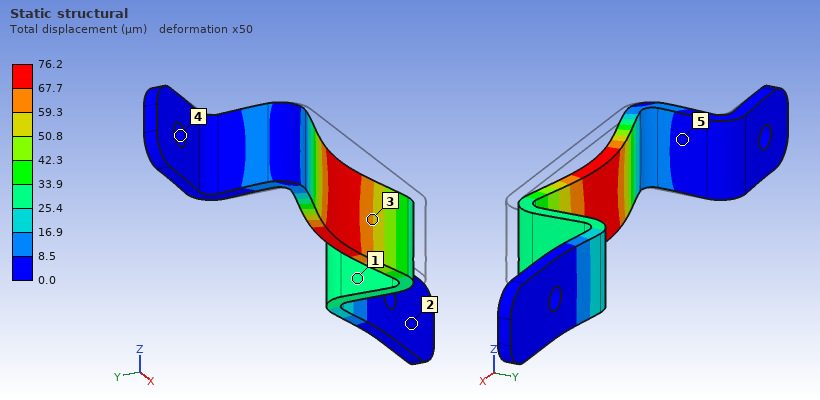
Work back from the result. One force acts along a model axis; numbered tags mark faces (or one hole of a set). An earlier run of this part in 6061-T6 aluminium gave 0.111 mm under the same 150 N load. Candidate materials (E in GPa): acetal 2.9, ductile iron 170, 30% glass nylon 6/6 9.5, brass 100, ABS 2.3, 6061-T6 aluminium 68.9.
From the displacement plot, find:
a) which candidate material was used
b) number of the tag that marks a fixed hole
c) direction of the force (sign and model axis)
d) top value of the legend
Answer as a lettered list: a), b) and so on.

a) brass
b) 4
c) +Y
d) 76.2 µm
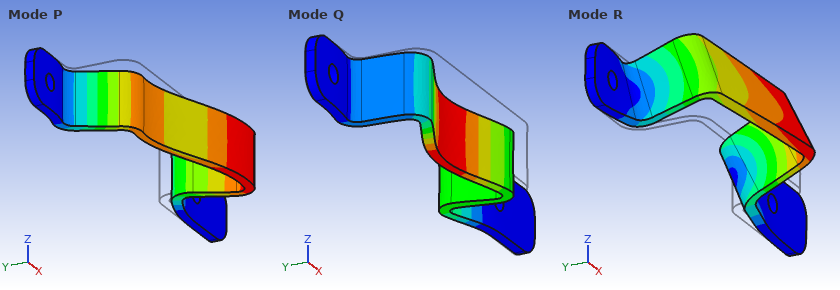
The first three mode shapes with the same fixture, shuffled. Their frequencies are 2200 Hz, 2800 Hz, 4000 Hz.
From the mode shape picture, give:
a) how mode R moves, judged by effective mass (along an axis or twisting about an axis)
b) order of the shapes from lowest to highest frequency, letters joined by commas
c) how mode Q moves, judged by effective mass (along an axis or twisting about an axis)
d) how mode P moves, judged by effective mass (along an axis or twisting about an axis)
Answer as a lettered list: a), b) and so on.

a) along Z
b) R, P, Q
c) along Y
d) along X
